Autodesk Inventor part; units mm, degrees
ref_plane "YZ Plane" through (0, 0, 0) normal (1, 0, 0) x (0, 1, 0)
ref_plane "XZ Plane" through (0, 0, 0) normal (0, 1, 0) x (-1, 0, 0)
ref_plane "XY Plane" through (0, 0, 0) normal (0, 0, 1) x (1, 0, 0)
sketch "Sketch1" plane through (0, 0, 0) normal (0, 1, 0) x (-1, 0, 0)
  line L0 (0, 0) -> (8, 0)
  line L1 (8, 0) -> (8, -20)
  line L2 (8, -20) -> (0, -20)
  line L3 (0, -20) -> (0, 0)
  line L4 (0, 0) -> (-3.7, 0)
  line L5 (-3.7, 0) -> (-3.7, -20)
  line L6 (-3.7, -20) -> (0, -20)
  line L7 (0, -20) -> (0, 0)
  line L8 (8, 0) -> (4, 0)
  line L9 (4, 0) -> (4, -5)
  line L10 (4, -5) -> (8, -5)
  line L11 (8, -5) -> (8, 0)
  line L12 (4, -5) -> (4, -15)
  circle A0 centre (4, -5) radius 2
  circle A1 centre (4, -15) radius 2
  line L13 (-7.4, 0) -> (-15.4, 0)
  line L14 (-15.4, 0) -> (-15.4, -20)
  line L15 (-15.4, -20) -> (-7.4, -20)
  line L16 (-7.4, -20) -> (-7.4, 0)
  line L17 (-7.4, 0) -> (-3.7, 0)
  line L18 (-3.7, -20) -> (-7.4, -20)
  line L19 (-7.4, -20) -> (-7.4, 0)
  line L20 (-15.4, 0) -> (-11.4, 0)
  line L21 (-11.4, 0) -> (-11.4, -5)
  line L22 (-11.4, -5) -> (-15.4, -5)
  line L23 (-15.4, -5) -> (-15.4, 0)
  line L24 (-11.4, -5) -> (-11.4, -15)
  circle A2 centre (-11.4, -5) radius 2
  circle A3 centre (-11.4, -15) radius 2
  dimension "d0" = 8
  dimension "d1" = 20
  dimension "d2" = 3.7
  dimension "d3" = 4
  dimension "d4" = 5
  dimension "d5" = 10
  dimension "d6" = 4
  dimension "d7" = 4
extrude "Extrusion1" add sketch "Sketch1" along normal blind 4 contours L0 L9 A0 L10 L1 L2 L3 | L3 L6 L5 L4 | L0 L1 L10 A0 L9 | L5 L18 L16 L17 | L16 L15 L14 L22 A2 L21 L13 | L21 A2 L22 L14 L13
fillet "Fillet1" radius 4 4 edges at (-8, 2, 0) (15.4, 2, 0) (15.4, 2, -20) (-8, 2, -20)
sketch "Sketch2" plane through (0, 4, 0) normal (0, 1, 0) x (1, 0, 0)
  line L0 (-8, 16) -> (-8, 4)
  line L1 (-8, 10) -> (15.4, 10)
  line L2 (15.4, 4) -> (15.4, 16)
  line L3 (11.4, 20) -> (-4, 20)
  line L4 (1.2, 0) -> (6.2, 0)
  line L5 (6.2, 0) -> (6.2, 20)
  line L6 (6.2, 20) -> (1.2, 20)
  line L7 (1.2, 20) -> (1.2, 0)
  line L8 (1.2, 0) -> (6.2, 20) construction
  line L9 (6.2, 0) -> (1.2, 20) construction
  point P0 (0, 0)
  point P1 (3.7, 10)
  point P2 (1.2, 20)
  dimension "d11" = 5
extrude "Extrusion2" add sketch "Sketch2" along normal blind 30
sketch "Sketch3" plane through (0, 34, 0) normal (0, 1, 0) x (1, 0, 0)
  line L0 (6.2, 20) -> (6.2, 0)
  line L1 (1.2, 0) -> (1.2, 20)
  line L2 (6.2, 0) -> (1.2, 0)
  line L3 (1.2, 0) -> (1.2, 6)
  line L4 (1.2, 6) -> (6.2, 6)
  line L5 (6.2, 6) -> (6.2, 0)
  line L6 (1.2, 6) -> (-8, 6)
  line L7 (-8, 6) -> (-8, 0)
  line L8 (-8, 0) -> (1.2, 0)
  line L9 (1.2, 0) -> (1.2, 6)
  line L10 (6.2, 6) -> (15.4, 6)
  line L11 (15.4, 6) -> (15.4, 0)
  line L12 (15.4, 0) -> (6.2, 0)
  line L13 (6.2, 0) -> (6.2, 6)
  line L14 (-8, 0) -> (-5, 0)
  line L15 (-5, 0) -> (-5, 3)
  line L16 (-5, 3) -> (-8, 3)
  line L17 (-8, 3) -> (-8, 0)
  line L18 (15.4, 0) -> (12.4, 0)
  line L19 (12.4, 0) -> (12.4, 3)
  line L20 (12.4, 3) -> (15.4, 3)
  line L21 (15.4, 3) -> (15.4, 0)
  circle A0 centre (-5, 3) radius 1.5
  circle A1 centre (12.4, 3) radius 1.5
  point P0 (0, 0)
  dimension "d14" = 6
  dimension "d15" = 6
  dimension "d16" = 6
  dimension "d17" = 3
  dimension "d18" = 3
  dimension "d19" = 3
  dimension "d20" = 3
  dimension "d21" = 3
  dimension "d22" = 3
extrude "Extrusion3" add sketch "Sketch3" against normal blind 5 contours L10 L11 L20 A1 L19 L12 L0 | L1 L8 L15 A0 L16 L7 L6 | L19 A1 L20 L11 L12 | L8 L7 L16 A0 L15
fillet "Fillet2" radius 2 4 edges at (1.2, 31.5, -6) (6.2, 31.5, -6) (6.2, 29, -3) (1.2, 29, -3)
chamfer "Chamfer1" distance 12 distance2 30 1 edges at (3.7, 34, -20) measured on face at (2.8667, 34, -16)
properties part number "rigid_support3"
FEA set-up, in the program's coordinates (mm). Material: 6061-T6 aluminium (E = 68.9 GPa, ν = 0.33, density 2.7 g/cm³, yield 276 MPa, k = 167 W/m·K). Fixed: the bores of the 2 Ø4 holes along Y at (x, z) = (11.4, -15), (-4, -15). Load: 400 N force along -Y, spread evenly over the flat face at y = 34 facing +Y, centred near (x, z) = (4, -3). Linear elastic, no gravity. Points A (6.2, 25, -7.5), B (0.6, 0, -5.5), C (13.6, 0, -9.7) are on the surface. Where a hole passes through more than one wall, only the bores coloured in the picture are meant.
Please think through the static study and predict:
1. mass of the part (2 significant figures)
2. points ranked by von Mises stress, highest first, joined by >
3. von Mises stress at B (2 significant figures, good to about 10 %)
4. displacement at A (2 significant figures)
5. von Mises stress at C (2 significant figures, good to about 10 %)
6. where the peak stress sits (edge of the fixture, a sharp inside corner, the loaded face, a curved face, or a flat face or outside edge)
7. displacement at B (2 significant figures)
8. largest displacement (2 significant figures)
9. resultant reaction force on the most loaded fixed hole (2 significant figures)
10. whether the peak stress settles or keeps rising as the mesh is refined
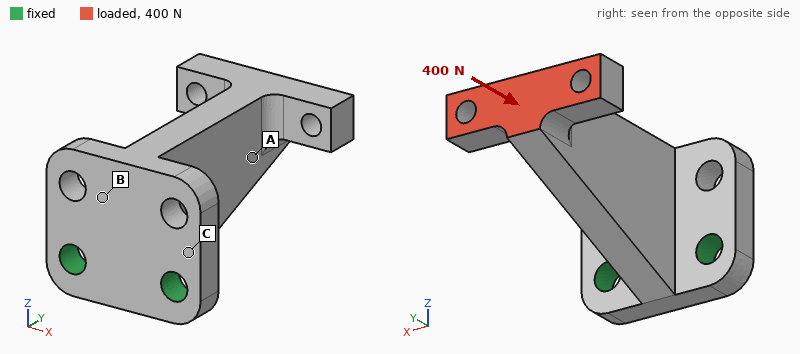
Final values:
11 g
C > B > A
15 MPa
40 µm
25 MPa
edge of the fixture
15 µm
65 µm
200 N
keeps rising
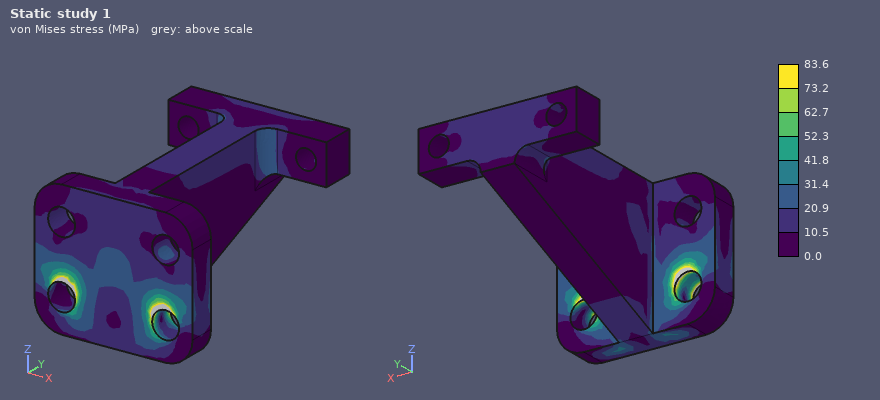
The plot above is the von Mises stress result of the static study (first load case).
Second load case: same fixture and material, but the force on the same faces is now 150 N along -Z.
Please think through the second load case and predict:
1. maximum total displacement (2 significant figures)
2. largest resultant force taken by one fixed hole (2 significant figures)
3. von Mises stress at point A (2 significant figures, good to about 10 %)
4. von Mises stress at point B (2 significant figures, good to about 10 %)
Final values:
74 µm
75 N
6.8 MPa
14 MPa
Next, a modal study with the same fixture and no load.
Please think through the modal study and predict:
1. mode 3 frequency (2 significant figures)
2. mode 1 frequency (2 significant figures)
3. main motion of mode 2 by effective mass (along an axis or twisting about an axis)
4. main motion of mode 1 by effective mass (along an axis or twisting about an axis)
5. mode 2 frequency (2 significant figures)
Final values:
11 kHz
3200 Hz
along Z
along X
4300 Hz
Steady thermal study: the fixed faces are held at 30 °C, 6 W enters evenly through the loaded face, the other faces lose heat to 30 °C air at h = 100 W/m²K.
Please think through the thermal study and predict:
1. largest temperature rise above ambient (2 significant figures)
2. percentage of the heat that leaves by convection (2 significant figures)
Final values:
16 K
25 %
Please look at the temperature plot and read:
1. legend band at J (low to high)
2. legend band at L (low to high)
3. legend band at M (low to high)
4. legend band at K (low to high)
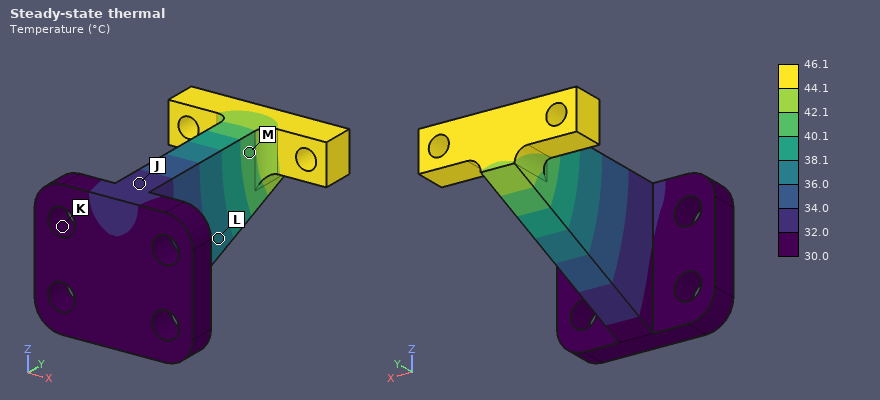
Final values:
32.0 to 34.0 °C
36.0 to 38.1 °C
40.1 to 42.1 °C
30.0 to 32.0 °C
